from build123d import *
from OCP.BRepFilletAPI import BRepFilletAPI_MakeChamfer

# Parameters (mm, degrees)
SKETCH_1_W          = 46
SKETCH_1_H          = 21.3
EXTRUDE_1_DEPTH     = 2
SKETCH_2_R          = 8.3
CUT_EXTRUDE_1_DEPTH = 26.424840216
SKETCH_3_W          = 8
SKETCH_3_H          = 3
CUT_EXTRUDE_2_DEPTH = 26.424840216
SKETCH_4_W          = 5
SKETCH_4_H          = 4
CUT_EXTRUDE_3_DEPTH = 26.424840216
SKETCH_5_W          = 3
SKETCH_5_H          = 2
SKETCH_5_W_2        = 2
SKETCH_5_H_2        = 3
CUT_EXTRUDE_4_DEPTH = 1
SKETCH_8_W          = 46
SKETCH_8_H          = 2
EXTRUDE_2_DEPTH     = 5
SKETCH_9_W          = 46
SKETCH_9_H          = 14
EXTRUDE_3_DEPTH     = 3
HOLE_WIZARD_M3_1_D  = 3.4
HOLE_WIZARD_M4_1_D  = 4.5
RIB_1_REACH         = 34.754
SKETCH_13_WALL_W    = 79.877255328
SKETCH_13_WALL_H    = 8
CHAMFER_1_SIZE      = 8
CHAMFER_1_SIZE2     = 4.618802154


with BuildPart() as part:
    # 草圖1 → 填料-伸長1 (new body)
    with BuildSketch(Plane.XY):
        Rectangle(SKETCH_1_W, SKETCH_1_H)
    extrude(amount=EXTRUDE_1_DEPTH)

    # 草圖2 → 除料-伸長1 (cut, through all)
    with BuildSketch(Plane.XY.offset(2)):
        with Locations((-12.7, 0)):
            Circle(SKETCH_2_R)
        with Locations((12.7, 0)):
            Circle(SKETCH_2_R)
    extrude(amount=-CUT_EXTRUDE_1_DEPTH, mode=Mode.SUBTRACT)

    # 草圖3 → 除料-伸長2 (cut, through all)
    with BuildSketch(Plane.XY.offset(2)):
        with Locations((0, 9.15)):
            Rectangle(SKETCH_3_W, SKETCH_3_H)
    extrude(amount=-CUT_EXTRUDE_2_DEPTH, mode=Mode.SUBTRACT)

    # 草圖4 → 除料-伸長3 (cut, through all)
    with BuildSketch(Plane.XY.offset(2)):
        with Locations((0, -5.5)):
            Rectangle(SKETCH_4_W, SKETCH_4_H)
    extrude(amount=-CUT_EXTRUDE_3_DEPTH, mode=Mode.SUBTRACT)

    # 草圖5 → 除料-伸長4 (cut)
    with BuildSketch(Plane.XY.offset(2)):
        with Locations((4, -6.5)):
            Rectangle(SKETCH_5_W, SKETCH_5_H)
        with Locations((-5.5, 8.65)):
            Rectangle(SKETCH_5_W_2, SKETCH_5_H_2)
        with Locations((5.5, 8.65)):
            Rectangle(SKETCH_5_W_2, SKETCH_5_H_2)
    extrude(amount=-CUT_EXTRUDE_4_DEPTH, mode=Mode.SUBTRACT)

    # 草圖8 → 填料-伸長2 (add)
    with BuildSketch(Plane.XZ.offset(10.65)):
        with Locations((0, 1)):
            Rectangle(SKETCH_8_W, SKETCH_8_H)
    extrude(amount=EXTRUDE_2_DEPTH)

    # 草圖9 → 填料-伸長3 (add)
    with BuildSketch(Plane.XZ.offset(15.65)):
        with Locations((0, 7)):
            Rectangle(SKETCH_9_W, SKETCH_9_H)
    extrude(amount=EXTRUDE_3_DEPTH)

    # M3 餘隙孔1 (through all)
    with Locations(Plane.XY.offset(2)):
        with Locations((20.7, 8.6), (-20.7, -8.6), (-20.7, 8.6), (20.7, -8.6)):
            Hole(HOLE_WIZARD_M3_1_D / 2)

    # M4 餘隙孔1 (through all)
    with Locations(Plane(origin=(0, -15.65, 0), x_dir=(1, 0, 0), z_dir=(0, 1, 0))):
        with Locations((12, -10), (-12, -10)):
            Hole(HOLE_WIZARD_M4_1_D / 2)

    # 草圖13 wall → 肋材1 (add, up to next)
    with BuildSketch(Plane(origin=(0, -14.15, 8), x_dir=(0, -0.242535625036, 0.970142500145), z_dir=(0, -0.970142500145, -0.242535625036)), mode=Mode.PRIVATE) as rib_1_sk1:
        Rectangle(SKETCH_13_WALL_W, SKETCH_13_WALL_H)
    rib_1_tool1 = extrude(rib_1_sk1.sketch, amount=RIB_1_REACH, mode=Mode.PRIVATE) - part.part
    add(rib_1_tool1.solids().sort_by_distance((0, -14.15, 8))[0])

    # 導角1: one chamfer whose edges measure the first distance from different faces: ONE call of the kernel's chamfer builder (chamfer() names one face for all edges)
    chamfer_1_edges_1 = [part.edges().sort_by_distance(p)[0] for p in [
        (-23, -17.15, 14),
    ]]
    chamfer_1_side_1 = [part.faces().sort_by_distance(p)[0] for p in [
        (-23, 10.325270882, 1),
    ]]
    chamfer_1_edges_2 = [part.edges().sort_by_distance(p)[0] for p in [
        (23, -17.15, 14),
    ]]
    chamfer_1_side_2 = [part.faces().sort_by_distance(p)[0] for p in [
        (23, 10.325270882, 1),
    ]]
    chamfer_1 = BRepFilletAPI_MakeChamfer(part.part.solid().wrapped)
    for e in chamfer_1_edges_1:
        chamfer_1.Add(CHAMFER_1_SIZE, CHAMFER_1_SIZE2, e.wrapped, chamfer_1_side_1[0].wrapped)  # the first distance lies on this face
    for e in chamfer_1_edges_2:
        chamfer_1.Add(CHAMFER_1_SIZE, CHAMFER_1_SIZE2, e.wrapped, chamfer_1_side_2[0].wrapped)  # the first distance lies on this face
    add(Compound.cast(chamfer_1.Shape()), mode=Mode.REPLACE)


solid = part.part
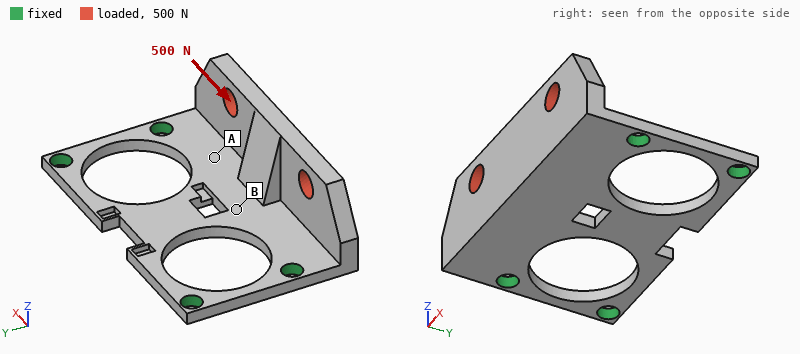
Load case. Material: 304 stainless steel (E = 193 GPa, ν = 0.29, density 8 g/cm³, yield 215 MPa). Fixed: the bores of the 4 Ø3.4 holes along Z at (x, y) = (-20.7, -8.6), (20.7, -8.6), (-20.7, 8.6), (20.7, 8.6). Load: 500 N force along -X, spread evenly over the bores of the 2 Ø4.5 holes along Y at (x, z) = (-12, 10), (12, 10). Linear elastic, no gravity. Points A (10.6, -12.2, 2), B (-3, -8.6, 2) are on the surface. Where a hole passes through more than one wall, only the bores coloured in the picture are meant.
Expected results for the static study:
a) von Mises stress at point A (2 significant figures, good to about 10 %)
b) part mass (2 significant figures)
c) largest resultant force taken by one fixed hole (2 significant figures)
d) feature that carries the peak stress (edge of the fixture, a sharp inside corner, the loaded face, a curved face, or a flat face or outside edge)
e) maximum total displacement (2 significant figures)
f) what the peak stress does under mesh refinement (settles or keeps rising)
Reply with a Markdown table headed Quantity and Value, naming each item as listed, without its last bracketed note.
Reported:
| Quantity | Value |
|---|---|
| von Mises stress at point A | 23 MPa |
| part mass | 26 g |
| largest resultant force taken by one fixed hole | 280 N |
| feature that carries the peak stress | edge of the fixture |
| maximum total displacement | 10 µm |
| what the peak stress does under mesh refinement | keeps rising |
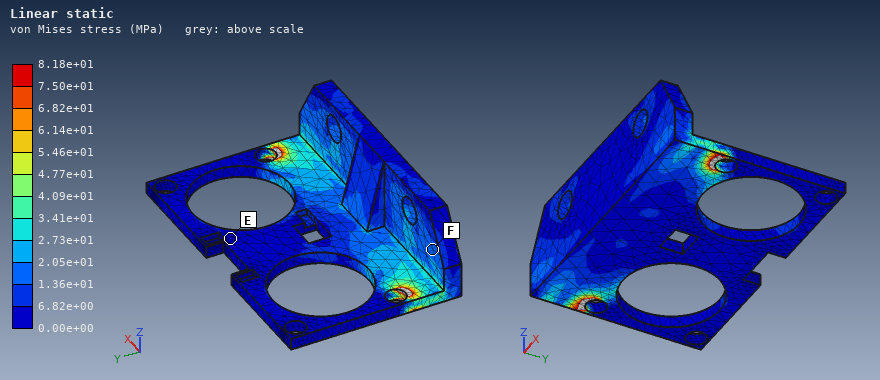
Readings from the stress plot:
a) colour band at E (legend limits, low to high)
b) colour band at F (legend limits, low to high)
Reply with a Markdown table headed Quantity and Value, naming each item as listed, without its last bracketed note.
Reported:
| Quantity | Value |
|---|---|
| colour band at E | 0.00e+00 to 6.82e+00 MPa |
| colour band at F | 1.36e+01 to 2.05e+01 MPa |
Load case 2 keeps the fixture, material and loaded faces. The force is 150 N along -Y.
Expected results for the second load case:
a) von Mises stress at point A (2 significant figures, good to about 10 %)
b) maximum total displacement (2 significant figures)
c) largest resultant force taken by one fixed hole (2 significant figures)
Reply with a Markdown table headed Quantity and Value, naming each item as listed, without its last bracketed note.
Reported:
| Quantity | Value |
|---|---|
| von Mises stress at point A | 31 MPa |
| maximum total displacement | 39 µm |
| largest resultant force taken by one fixed hole | 89 N |
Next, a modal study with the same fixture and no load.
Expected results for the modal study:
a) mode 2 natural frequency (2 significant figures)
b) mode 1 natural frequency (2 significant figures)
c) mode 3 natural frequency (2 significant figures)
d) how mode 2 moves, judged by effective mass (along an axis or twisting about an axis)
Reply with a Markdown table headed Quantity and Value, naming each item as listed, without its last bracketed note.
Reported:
| Quantity | Value |
|---|---|
| mode 2 natural frequency | 6400 Hz |
| mode 1 natural frequency | 3400 Hz |
| mode 3 natural frequency | 9000 Hz |
| how mode 2 moves, judged by effective mass | along Z |
